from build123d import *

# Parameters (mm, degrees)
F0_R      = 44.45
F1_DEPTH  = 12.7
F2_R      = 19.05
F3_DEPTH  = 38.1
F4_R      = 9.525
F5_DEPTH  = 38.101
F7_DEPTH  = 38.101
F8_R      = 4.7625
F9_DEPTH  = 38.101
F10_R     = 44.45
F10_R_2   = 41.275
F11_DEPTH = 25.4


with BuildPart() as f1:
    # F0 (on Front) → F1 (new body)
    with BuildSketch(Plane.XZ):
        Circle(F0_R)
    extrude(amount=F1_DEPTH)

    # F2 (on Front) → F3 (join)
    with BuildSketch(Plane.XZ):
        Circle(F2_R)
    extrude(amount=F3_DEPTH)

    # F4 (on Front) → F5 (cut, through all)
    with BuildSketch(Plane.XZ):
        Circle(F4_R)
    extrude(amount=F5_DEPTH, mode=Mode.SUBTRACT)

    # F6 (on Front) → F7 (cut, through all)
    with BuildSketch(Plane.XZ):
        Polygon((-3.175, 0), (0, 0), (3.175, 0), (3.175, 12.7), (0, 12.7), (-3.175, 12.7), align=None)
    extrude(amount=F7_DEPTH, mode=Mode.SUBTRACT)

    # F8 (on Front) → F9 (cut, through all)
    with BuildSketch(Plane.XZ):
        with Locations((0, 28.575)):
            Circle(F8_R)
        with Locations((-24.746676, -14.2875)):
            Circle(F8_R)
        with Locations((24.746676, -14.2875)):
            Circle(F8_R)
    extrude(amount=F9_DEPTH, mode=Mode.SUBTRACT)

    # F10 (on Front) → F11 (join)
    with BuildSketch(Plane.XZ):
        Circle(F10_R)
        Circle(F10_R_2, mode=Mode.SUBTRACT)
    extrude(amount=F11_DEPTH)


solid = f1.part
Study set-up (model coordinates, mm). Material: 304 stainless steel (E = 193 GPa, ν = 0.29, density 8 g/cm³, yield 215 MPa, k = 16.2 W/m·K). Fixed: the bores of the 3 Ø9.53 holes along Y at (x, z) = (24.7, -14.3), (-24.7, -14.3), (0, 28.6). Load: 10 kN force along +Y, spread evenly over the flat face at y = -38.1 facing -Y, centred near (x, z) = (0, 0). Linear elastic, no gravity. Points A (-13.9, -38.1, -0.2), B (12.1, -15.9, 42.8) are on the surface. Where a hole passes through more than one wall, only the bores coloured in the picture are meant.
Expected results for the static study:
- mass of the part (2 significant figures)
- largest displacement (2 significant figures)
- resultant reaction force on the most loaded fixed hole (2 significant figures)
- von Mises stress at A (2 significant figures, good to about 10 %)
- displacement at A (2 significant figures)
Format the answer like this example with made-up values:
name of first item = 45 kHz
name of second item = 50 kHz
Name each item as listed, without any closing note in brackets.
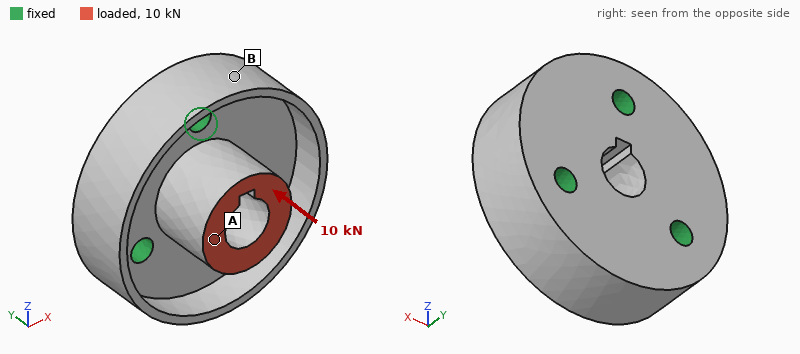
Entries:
mass of the part = 830 g
largest displacement = 4.0 µm
resultant reaction force on the most loaded fixed hole = 3.5 kN
von Mises stress at A = 13 MPa
displacement at A = 3.9 µm
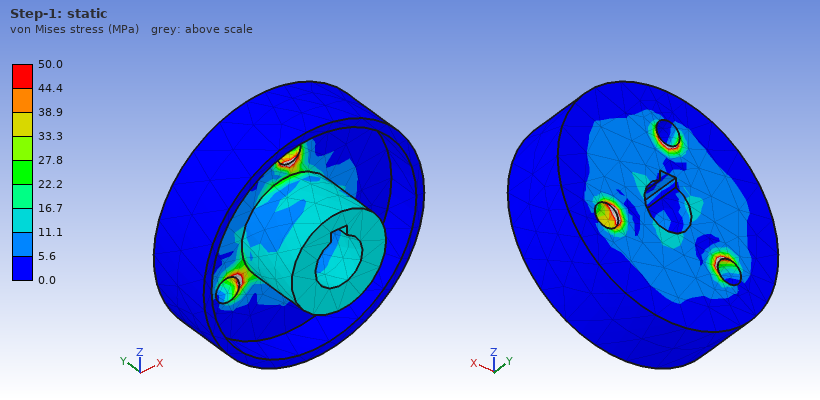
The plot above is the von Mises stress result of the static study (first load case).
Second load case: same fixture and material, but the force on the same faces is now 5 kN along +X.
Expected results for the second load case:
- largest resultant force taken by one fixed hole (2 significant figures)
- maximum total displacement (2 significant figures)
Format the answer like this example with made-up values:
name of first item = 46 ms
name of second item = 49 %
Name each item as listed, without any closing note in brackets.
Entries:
largest resultant force taken by one fixed hole = 3.6 kN
maximum total displacement = 11 µm
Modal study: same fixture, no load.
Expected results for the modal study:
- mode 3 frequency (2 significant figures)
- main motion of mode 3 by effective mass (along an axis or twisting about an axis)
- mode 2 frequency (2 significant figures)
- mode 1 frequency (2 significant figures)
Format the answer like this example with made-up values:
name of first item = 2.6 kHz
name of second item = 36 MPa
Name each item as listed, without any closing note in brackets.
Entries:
mode 3 frequency = 11 kHz
main motion of mode 3 by effective mass = along Y
mode 2 frequency = 9300 Hz
mode 1 frequency = 9300 Hz
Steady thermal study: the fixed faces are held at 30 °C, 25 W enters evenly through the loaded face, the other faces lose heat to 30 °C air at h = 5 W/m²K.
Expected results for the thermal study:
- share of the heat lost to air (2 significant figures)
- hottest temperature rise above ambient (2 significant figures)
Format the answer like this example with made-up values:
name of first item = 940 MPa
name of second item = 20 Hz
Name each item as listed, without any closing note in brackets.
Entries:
share of the heat lost to air = 6.5 %
hottest temperature rise above ambient = 65 K
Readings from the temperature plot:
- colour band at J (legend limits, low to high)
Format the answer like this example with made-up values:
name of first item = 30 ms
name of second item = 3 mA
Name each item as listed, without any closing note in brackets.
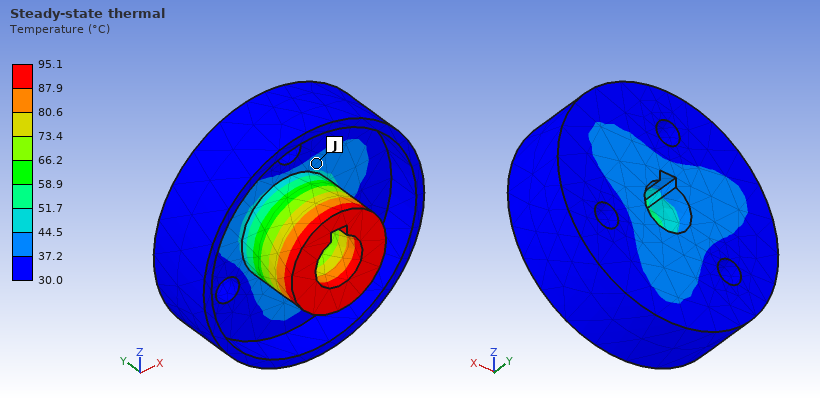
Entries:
colour band at J = 37.2 to 44.5 °C
